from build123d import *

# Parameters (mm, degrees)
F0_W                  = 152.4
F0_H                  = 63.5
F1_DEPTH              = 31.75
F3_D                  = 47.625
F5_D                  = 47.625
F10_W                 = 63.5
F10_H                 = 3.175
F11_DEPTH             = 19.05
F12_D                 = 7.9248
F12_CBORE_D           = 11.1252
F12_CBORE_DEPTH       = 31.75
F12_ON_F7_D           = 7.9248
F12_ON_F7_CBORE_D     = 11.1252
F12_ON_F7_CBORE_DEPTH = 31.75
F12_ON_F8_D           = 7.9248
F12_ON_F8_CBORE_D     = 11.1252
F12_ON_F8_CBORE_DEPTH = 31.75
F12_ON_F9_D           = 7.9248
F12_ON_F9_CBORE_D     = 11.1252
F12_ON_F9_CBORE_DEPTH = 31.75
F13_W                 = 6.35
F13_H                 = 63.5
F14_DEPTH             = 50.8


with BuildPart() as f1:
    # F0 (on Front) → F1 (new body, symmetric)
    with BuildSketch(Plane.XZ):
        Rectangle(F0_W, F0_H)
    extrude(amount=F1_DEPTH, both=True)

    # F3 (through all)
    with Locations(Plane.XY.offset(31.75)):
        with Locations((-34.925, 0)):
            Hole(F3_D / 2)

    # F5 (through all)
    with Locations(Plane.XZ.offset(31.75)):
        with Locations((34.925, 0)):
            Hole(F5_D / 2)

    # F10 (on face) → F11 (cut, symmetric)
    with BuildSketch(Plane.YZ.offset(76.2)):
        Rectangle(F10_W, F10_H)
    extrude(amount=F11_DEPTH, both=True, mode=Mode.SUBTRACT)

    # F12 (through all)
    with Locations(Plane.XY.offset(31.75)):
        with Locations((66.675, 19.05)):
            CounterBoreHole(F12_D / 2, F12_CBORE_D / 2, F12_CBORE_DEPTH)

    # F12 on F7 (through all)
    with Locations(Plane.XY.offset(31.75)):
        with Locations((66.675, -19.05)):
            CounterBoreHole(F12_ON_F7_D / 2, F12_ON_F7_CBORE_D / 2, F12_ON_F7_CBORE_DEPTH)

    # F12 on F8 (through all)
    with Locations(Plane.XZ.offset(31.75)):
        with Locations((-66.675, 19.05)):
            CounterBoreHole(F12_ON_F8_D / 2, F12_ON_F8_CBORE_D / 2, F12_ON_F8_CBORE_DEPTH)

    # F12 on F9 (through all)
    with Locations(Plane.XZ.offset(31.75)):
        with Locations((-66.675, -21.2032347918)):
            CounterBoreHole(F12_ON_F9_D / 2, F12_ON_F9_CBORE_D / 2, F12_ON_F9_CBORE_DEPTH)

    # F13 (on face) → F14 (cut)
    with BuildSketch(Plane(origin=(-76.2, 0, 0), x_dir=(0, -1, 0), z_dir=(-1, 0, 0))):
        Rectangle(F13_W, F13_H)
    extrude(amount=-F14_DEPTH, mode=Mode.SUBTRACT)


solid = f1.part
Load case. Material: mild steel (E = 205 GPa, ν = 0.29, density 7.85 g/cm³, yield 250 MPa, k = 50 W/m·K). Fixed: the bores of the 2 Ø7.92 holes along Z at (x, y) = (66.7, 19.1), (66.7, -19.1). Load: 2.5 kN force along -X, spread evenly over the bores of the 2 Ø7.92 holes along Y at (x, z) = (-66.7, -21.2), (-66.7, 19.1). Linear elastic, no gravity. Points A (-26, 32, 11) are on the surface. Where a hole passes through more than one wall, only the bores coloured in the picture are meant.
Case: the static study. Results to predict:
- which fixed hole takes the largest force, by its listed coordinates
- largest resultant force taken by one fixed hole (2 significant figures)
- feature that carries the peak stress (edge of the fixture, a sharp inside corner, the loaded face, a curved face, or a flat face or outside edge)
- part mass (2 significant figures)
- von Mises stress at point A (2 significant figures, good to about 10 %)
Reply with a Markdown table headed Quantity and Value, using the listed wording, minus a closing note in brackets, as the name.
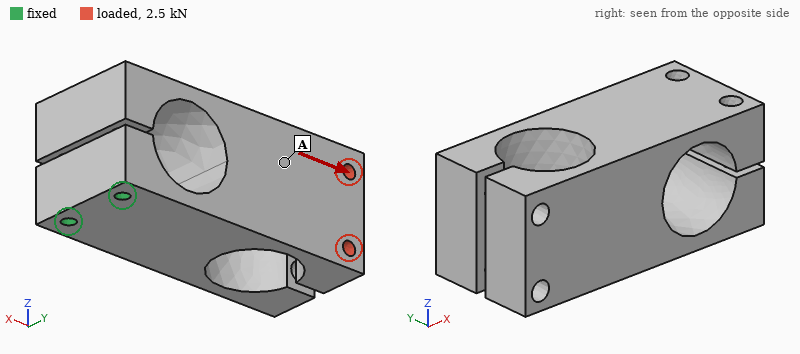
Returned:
| Quantity | Value |
|---|---|
| which fixed hole takes the largest force, by its listed coordinates | (66.7, 19.1) |
| largest resultant force taken by one fixed hole | 2.3 kN |
| feature that carries the peak stress | a curved face |
| part mass | 2.8 kg |
| von Mises stress at point A | 19 MPa |
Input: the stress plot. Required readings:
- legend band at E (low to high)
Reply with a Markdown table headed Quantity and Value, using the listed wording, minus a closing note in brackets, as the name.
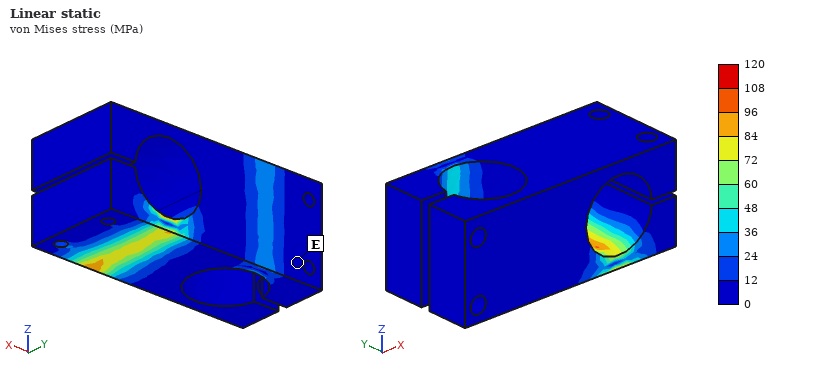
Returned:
| Quantity | Value |
|---|---|
| legend band at E | 0 to 12 MPa |
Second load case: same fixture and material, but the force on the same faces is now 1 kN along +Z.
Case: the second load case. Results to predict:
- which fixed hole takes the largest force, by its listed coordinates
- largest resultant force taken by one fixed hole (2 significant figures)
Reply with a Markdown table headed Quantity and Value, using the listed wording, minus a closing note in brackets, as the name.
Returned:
| Quantity | Value |
|---|---|
| which fixed hole takes the largest force, by its listed coordinates | (66.7, 19.1) |
| largest resultant force taken by one fixed hole | 850 N |
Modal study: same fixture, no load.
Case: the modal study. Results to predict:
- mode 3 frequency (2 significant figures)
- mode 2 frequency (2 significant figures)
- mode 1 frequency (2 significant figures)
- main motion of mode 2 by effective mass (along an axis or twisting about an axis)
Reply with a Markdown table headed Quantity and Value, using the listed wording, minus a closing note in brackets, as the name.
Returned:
| Quantity | Value |
|---|---|
| mode 3 frequency | 1000 Hz |
| mode 2 frequency | 660 Hz |
| mode 1 frequency | 220 Hz |
| main motion of mode 2 by effective mass | along Y |
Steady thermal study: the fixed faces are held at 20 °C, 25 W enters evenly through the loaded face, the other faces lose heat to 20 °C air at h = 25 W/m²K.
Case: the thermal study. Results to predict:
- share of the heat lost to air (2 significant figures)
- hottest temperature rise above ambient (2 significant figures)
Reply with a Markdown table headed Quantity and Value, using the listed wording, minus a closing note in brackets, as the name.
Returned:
| Quantity | Value |
|---|---|
| share of the heat lost to air | 77 % |
| hottest temperature rise above ambient | 43 K |
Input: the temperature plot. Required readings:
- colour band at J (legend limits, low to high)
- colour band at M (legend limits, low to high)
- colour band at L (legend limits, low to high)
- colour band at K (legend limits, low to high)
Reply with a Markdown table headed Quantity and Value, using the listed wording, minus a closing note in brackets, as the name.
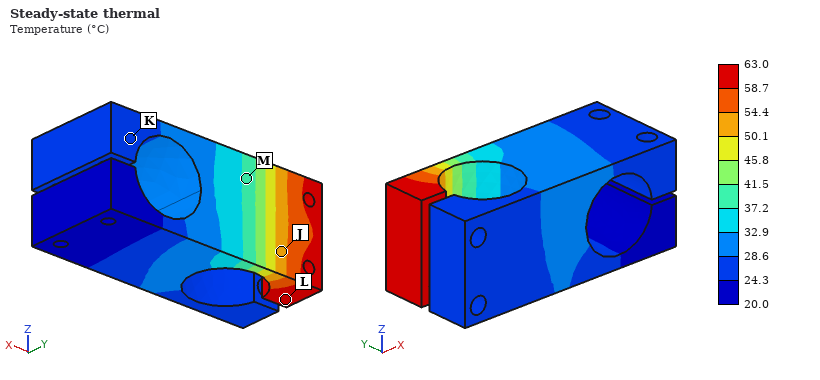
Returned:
| Quantity | Value |
|---|---|
| colour band at J | 50.1 to 54.4 °C |
| colour band at M | 37.2 to 41.5 °C |
| colour band at L | 58.7 to 63.0 °C |
| colour band at K | 24.3 to 28.6 °C |
